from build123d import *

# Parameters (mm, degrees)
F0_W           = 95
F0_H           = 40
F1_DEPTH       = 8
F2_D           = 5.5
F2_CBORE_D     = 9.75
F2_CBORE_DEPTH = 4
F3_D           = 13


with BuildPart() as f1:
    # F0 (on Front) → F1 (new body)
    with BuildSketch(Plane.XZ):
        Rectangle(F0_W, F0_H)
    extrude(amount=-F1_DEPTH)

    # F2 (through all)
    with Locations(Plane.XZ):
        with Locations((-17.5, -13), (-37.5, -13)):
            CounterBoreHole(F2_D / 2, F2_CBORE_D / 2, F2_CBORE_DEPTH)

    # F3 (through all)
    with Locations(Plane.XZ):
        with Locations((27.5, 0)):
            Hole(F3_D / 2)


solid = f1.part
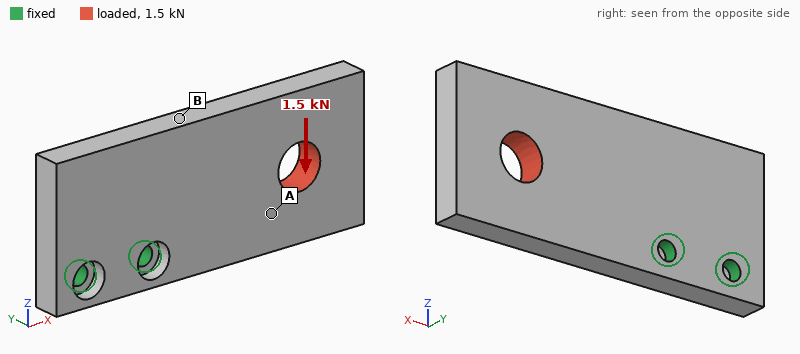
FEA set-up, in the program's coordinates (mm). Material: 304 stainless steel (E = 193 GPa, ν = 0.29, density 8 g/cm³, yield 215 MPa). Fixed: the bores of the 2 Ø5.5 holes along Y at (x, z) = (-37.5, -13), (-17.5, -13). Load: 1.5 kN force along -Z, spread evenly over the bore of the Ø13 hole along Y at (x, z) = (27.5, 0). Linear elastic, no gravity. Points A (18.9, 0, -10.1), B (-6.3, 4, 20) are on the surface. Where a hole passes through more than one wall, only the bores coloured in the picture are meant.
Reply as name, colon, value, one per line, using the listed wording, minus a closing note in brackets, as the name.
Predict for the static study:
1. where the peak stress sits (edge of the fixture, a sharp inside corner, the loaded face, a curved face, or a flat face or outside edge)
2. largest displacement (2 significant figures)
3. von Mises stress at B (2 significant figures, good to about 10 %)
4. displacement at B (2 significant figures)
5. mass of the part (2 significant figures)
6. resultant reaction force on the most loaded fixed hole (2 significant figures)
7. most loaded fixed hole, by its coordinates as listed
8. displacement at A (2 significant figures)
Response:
where the peak stress sits: edge of the fixture
largest displacement: 47 µm
von Mises stress at B: 26 MPa
displacement at B: 18 µm
mass of the part: 230 g
resultant reaction force on the most loaded fixed hole: 4.2 kN
most loaded fixed hole, by its coordinates as listed: (-17.5, -13)
displacement at A: 24 µm
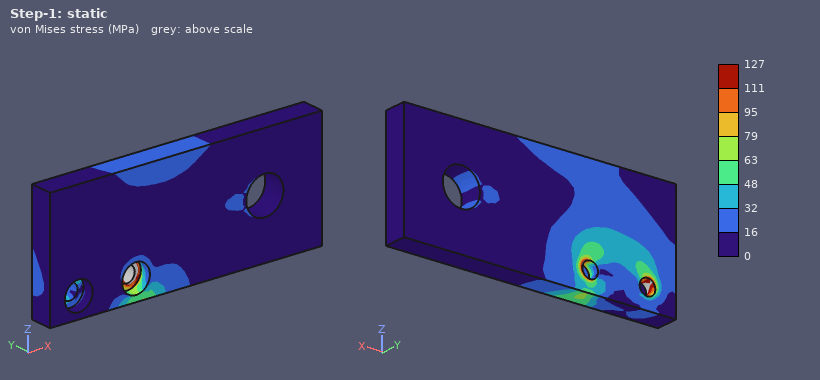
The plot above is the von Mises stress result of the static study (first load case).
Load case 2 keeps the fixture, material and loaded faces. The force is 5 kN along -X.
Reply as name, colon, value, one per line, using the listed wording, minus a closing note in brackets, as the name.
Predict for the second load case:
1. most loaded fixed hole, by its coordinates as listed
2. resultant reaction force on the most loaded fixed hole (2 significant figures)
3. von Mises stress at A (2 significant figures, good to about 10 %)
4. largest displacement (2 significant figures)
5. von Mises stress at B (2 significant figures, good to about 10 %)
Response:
most loaded fixed hole, by its coordinates as listed: (-17.5, -13)
resultant reaction force on the most loaded fixed hole: 4.1 kN
von Mises stress at A: 20 MPa
largest displacement: 25 µm
von Mises stress at B: 18 MPa
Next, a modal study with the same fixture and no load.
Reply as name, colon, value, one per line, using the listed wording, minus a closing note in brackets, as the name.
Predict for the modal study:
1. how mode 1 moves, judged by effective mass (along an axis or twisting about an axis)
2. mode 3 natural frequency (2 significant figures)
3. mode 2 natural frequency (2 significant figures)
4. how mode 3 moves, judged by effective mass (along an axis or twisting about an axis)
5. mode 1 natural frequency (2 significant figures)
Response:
how mode 1 moves, judged by effective mass: along Y
mode 3 natural frequency: 3400 Hz
mode 2 natural frequency: 2700 Hz
how mode 3 moves, judged by effective mass: along Z
mode 1 natural frequency: 1100 Hz
